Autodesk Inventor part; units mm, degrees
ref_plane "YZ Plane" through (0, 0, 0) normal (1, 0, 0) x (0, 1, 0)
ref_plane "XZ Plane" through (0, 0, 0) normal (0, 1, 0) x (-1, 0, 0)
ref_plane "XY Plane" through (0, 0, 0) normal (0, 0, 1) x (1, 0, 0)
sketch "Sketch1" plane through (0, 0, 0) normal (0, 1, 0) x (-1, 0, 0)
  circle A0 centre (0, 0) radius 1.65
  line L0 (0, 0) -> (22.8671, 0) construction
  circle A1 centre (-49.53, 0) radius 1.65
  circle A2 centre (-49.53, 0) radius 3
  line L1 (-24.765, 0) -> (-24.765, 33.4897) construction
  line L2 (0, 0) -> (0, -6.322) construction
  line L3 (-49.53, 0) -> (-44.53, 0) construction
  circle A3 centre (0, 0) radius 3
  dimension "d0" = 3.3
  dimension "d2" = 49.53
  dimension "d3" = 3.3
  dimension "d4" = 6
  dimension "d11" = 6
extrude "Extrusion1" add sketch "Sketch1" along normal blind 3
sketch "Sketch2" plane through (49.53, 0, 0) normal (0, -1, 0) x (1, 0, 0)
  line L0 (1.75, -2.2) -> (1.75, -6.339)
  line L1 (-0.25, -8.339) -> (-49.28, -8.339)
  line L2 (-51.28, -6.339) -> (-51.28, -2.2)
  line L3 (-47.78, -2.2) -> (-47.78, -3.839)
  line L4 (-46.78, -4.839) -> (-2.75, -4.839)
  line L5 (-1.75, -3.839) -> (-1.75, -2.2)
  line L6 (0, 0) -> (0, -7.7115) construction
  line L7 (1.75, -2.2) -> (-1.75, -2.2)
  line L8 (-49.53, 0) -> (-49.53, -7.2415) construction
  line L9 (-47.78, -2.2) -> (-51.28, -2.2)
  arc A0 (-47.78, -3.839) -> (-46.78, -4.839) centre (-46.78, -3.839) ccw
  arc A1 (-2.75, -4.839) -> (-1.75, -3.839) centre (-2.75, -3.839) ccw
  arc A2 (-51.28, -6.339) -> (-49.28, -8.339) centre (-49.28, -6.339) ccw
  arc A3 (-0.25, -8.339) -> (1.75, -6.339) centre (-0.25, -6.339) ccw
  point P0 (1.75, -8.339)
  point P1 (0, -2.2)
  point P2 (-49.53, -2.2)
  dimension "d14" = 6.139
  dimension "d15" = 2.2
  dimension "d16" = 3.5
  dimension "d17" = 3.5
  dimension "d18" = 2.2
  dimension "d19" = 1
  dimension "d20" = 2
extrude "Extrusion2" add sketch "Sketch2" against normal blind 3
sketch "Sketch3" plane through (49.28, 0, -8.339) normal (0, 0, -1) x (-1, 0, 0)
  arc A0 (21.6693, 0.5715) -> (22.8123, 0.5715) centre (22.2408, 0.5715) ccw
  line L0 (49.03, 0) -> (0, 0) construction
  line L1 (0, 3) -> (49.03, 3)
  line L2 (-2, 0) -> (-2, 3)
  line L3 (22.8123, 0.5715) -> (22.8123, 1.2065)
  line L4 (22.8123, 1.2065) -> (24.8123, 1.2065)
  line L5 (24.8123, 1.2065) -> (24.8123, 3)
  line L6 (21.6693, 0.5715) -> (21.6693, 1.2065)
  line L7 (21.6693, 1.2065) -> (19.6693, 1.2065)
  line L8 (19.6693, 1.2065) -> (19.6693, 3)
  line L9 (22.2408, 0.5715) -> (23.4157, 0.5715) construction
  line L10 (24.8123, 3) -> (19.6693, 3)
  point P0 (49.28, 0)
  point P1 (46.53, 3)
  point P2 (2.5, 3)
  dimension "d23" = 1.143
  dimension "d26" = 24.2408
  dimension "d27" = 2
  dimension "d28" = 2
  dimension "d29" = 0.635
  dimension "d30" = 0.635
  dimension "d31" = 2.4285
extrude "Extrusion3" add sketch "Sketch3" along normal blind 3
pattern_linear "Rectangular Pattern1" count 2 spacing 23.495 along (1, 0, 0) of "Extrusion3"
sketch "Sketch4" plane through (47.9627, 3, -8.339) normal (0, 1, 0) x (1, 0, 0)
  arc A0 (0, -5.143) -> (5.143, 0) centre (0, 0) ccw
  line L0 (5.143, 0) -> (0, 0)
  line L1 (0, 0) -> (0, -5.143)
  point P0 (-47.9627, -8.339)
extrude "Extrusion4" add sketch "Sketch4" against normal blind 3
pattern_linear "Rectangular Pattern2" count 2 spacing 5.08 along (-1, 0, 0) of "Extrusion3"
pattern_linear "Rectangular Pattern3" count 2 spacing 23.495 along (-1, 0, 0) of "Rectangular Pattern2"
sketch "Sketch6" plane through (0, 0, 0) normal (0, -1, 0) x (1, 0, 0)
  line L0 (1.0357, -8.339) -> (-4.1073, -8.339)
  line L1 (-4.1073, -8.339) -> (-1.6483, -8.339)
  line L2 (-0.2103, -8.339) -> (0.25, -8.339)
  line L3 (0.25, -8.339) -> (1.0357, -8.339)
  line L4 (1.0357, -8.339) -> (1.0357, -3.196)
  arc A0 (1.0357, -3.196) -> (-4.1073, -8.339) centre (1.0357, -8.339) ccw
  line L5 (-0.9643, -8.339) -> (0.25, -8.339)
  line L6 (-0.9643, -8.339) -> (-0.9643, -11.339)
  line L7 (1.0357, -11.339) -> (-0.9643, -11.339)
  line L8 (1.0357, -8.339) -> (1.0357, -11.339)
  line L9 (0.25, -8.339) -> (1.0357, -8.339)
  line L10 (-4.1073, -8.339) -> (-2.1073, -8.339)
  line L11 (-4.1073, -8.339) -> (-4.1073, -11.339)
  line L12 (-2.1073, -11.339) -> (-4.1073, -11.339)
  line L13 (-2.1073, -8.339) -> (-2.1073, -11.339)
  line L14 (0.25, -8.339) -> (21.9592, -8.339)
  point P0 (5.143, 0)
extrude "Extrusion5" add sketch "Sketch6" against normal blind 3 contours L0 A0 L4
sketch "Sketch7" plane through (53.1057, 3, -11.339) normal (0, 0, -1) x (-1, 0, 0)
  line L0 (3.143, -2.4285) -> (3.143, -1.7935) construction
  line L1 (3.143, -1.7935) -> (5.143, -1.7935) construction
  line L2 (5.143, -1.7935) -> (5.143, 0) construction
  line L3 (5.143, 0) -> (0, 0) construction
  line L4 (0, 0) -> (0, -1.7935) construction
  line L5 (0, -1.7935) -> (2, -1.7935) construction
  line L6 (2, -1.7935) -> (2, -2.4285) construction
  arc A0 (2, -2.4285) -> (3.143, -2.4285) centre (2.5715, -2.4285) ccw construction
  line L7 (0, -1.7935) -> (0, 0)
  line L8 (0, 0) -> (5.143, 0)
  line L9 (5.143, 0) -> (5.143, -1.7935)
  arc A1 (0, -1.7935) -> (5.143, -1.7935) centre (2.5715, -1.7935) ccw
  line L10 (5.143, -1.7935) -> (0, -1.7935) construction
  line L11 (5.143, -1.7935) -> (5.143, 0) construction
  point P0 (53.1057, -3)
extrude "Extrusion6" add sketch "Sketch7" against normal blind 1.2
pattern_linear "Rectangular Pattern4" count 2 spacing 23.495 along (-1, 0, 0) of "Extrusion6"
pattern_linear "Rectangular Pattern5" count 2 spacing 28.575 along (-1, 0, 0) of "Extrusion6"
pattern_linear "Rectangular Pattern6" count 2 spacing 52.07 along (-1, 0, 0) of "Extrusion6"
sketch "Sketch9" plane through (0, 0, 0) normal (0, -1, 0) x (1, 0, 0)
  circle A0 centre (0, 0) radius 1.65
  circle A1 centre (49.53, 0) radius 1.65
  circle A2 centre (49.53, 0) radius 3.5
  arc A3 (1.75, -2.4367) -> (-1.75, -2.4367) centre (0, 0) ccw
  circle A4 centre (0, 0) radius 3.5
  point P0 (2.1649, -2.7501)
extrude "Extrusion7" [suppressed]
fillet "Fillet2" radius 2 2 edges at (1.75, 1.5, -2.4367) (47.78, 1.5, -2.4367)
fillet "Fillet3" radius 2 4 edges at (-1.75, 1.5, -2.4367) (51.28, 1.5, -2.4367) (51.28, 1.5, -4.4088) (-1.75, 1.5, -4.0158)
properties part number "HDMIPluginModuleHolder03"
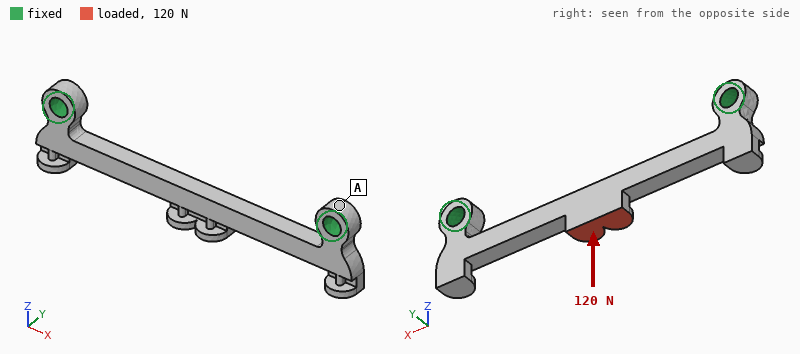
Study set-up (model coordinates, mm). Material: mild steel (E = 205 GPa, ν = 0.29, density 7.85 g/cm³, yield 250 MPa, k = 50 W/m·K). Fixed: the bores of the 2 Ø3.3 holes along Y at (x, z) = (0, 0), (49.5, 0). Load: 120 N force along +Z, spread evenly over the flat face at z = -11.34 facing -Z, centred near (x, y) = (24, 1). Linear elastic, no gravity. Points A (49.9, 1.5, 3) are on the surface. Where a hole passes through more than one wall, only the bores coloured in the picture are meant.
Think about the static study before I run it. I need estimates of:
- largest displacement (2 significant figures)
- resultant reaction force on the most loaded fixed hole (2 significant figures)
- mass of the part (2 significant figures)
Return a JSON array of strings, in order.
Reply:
["30 µm", "130 N", "7.3 g"]
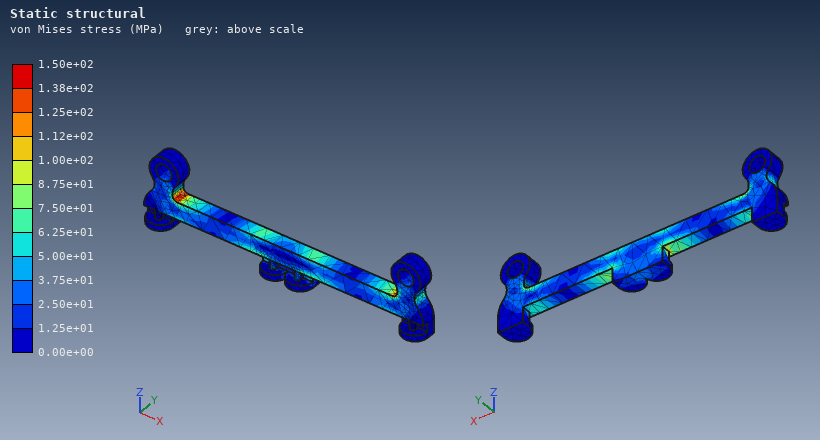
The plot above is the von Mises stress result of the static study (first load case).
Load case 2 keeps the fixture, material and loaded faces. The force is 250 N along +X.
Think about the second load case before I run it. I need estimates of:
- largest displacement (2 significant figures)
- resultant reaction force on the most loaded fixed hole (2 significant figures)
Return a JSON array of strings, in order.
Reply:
["9.4 µm", "130 N"]
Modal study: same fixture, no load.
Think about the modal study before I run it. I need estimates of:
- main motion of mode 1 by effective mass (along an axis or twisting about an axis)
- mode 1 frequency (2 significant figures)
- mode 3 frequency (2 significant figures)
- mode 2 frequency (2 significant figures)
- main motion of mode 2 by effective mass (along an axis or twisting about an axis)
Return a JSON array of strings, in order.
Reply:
["along Y", "4400 Hz", "13 kHz", "6600 Hz", "along Z"]
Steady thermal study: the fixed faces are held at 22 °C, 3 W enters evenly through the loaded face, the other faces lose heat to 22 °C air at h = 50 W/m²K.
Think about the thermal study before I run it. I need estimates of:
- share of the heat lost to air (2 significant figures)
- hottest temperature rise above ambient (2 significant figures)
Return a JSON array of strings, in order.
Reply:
["41 %", "59 K"]
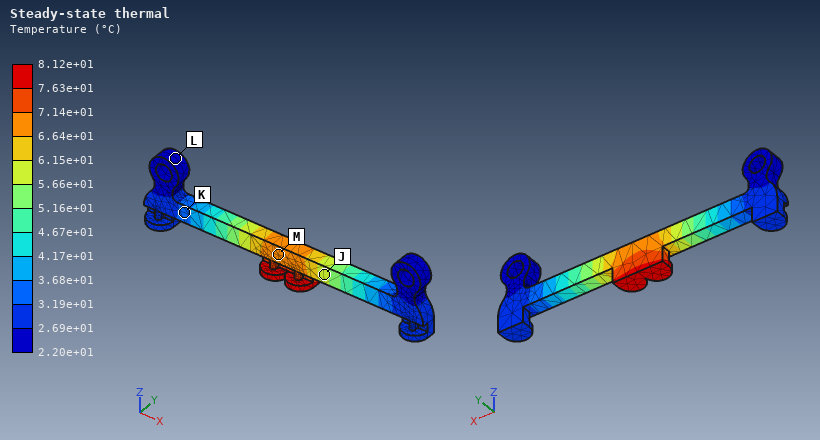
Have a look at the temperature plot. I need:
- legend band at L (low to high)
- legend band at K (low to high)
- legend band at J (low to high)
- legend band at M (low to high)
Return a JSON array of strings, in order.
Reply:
["2.20e+01 to 2.69e+01 °C", "3.19e+01 to 3.68e+01 °C", "5.66e+01 to 6.15e+01 °C", "6.64e+01 to 7.14e+01 °C"]
